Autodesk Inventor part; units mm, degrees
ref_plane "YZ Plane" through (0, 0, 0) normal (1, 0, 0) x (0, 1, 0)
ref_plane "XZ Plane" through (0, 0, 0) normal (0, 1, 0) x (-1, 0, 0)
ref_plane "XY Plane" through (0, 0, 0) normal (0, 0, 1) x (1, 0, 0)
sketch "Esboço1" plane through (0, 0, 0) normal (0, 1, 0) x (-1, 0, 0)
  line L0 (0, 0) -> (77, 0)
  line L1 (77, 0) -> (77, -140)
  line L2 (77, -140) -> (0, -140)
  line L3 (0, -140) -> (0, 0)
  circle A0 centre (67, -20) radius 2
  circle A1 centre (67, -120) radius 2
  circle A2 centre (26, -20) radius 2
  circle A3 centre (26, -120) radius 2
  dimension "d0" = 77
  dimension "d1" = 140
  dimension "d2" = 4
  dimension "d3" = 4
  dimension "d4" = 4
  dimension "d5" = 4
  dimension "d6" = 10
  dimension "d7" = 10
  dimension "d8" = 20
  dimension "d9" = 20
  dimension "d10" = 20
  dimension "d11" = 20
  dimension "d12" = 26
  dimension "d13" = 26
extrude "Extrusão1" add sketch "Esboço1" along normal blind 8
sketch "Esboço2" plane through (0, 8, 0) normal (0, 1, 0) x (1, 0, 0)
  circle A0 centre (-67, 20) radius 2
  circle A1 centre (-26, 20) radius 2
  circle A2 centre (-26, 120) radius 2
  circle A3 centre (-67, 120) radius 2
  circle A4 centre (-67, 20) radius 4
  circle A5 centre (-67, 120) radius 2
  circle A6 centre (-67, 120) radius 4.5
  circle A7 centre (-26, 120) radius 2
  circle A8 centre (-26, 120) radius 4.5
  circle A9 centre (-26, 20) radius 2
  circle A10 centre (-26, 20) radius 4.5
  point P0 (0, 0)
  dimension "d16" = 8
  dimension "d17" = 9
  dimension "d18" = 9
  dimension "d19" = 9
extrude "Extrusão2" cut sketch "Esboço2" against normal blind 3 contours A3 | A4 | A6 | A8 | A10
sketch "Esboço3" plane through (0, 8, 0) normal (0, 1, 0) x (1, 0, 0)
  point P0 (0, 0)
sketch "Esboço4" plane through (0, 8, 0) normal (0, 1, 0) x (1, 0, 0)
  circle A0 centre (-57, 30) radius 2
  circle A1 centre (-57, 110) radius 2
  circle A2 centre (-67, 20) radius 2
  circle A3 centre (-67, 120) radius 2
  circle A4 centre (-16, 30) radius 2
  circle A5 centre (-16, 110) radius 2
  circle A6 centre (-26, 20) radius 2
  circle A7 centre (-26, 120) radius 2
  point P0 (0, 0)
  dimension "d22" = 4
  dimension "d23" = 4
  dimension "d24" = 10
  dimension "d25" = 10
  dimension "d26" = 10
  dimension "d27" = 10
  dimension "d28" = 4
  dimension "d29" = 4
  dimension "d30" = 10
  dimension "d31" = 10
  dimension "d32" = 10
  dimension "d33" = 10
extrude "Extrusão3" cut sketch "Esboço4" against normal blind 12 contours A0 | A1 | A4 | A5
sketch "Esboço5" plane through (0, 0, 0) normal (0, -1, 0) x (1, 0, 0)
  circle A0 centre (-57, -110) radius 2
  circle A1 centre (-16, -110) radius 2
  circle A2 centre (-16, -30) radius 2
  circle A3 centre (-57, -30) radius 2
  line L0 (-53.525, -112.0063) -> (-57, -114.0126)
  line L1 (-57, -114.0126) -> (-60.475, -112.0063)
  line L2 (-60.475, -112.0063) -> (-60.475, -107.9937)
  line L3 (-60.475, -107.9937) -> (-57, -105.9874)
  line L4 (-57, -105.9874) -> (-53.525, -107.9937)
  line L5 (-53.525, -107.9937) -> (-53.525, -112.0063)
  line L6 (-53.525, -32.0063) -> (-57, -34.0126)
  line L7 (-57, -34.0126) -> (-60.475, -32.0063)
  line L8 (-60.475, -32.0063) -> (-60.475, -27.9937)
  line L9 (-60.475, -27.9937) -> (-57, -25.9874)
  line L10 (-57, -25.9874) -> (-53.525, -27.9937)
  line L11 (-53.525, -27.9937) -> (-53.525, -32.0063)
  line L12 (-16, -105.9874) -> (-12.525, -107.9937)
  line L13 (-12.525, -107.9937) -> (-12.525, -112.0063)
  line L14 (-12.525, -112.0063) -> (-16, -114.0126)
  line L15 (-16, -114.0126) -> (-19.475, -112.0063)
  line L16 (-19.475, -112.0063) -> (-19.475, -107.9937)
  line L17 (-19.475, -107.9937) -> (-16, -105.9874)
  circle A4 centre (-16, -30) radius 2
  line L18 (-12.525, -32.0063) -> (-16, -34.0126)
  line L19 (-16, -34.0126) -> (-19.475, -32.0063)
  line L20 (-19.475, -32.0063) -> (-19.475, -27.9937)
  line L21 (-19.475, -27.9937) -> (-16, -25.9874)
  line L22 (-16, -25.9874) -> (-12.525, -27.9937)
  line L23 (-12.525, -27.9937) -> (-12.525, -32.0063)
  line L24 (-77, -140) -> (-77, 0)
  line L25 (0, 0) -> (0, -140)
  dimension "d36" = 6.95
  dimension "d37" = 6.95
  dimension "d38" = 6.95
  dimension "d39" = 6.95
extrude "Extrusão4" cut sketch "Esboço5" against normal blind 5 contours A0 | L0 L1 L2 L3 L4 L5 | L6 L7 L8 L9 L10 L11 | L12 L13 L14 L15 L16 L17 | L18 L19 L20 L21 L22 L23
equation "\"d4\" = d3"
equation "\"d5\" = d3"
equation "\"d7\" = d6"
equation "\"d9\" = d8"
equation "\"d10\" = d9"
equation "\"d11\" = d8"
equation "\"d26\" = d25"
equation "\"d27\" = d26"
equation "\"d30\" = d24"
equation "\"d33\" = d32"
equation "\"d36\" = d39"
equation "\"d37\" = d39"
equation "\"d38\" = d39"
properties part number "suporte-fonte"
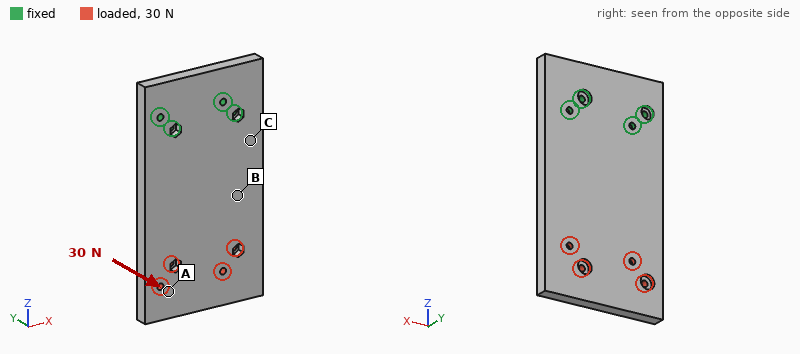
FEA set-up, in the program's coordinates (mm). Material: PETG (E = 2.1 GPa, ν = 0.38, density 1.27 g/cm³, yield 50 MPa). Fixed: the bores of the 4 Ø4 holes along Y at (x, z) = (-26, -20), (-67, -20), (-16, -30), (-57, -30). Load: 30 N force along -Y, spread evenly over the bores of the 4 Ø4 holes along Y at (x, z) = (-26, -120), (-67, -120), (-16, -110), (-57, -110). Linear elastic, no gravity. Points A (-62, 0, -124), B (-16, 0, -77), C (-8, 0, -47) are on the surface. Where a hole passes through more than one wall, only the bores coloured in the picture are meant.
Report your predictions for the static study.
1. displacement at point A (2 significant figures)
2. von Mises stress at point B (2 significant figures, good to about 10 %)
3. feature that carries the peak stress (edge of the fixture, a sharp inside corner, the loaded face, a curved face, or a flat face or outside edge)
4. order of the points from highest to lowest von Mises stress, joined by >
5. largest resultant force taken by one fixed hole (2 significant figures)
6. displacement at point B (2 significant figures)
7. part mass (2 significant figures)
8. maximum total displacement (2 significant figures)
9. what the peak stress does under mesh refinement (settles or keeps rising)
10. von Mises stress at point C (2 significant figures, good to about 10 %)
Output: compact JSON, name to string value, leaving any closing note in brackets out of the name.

{"displacement at point A": "1.3 mm", "von Mises stress at point B": "1.4 MPa", "feature that carries the peak stress": "edge of the fixture", "order of the points from highest to lowest von Mises stress, joined by >": "C > B > A", "largest resultant force taken by one fixed hole": "140 N", "displacement at point B": "0.47 mm", "part mass": "110 g", "maximum total displacement": "1.6 mm", "what the peak stress does under mesh refinement": "keeps rising", "von Mises stress at point C": "2.3 MPa"}
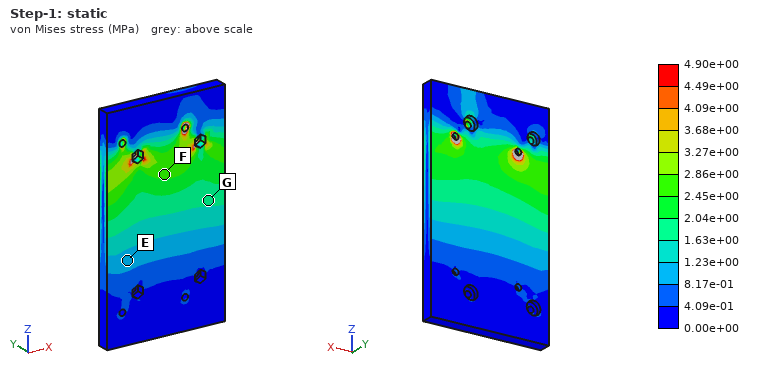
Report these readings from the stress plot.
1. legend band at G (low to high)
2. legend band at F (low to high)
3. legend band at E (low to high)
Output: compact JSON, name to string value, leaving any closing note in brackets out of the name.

{"legend band at G": "1.63e+00 to 2.04e+00 MPa", "legend band at F": "2.45e+00 to 2.86e+00 MPa", "legend band at E": "8.17e-01 to 1.23e+00 MPa"}
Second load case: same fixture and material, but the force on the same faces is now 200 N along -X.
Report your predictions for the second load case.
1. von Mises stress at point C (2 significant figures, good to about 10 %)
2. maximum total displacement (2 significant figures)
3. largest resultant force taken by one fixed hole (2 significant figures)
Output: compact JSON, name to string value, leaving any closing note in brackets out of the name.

{"von Mises stress at point C": "1.1 MPa", "maximum total displacement": "0.24 mm", "largest resultant force taken by one fixed hole": "260 N"}
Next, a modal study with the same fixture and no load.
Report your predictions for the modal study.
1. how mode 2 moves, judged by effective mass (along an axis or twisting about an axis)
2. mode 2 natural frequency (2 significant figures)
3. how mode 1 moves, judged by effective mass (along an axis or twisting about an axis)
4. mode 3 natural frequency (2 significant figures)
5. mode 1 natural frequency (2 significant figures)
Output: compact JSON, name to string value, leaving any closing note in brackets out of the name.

{"how mode 2 moves, judged by effective mass": "twisting about Z", "mode 2 natural frequency": "400 Hz", "how mode 1 moves, judged by effective mass": "along Y", "mode 3 natural frequency": "740 Hz", "mode 1 natural frequency": "120 Hz"}
